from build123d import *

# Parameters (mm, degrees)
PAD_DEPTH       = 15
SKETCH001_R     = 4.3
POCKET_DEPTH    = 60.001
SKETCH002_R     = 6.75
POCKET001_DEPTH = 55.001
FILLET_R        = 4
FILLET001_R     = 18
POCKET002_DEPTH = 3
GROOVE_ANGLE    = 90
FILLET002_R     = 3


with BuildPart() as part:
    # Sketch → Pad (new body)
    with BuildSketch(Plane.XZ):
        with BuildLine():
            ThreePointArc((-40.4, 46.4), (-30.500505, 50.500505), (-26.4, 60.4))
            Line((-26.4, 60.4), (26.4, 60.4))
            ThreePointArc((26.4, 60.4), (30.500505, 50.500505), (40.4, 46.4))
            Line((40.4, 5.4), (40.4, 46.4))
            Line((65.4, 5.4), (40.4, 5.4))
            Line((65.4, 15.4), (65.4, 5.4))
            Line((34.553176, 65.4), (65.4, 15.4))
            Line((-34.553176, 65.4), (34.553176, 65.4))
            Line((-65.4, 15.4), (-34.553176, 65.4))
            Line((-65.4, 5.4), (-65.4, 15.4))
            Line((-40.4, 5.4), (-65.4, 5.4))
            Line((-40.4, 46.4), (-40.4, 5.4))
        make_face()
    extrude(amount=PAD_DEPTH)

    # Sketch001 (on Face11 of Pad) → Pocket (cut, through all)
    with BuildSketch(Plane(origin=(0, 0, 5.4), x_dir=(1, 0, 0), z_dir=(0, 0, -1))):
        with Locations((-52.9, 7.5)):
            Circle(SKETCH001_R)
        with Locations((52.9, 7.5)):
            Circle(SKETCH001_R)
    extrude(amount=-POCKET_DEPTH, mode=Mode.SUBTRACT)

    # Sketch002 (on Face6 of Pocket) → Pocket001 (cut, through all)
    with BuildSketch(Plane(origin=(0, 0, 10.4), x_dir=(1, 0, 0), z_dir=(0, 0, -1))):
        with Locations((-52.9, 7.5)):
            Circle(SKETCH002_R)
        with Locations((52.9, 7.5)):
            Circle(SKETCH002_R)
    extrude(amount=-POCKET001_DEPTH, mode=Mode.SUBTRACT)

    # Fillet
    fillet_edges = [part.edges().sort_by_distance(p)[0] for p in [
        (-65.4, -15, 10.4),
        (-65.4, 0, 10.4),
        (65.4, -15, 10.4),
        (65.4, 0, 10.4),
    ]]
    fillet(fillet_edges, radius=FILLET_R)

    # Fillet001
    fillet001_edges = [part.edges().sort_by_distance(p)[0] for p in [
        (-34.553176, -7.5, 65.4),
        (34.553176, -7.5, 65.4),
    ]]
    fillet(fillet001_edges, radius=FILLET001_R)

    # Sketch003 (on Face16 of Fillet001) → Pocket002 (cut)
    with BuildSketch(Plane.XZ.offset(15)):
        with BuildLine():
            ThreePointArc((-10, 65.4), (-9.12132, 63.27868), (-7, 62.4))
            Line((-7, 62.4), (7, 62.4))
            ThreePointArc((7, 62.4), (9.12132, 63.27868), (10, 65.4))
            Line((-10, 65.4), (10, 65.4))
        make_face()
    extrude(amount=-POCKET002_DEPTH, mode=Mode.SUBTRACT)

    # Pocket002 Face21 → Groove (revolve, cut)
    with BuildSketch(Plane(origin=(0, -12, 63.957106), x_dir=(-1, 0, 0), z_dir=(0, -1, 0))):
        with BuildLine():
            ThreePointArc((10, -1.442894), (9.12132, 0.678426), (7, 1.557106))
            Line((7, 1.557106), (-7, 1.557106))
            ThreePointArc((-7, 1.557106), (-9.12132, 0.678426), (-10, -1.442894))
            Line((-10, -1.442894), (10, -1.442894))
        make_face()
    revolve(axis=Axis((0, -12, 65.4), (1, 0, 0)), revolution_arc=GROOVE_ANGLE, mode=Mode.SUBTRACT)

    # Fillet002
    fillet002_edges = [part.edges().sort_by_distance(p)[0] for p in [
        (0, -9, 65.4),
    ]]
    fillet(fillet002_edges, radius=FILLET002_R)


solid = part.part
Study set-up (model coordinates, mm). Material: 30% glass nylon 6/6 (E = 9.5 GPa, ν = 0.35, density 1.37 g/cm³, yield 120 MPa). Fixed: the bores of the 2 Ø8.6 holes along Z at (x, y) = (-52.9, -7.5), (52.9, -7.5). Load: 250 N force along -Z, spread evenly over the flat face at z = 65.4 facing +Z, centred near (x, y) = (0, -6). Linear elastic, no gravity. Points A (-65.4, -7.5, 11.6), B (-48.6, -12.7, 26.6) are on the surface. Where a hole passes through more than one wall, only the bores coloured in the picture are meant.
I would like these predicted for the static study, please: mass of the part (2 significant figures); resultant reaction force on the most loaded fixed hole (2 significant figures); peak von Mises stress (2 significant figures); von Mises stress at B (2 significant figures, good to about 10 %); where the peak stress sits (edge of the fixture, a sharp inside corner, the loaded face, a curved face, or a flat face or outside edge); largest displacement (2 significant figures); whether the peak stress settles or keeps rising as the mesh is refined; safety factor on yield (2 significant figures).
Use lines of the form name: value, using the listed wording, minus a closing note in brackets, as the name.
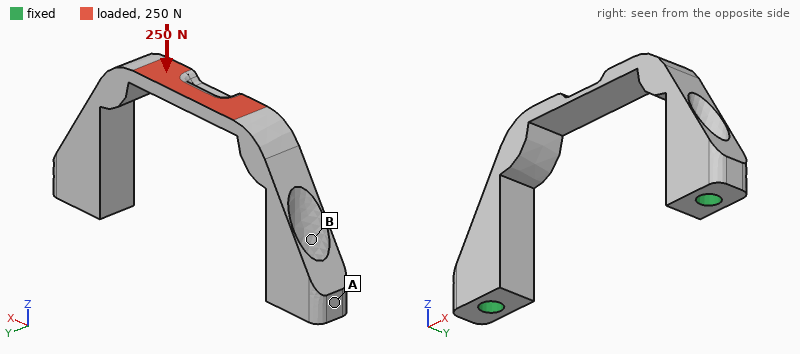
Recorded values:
mass of the part: 33 g
resultant reaction force on the most loaded fixed hole: 160 N
peak von Mises stress: 20 MPa
von Mises stress at B: 3.0 MPa
where the peak stress sits: the loaded face
largest displacement: 0.24 mm
whether the peak stress settles or keeps rising as the mesh is refined: settles
safety factor on yield: 5.9
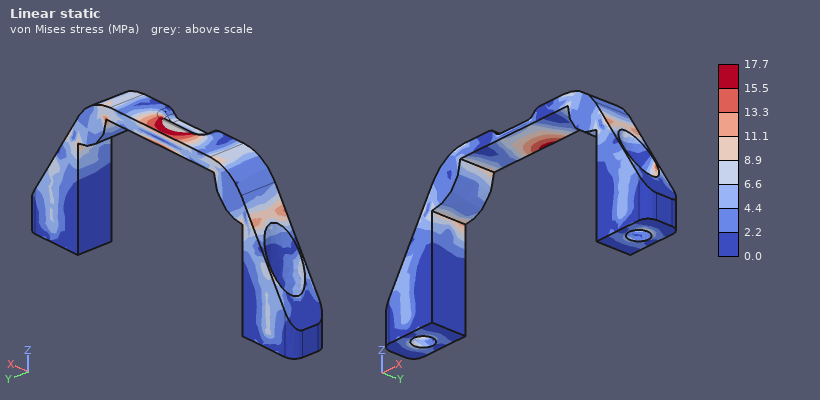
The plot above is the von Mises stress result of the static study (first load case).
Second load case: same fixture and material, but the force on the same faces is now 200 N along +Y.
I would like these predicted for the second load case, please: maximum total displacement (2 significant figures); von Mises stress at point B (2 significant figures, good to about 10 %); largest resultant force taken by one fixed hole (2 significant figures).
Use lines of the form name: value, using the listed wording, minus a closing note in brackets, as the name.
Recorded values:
maximum total displacement: 0.52 mm
von Mises stress at point B: 7.7 MPa
largest resultant force taken by one fixed hole: 100 N
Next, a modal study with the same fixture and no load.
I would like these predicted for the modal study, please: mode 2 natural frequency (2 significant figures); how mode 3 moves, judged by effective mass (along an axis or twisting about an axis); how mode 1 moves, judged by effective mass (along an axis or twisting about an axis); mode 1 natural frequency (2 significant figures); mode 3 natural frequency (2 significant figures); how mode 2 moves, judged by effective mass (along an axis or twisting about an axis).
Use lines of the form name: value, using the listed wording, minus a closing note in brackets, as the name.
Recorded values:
mode 2 natural frequency: 1400 Hz
how mode 3 moves, judged by effective mass: twisting about Z
how mode 1 moves, judged by effective mass: along Y
mode 1 natural frequency: 1100 Hz
mode 3 natural frequency: 1600 Hz
how mode 2 moves, judged by effective mass: along X
